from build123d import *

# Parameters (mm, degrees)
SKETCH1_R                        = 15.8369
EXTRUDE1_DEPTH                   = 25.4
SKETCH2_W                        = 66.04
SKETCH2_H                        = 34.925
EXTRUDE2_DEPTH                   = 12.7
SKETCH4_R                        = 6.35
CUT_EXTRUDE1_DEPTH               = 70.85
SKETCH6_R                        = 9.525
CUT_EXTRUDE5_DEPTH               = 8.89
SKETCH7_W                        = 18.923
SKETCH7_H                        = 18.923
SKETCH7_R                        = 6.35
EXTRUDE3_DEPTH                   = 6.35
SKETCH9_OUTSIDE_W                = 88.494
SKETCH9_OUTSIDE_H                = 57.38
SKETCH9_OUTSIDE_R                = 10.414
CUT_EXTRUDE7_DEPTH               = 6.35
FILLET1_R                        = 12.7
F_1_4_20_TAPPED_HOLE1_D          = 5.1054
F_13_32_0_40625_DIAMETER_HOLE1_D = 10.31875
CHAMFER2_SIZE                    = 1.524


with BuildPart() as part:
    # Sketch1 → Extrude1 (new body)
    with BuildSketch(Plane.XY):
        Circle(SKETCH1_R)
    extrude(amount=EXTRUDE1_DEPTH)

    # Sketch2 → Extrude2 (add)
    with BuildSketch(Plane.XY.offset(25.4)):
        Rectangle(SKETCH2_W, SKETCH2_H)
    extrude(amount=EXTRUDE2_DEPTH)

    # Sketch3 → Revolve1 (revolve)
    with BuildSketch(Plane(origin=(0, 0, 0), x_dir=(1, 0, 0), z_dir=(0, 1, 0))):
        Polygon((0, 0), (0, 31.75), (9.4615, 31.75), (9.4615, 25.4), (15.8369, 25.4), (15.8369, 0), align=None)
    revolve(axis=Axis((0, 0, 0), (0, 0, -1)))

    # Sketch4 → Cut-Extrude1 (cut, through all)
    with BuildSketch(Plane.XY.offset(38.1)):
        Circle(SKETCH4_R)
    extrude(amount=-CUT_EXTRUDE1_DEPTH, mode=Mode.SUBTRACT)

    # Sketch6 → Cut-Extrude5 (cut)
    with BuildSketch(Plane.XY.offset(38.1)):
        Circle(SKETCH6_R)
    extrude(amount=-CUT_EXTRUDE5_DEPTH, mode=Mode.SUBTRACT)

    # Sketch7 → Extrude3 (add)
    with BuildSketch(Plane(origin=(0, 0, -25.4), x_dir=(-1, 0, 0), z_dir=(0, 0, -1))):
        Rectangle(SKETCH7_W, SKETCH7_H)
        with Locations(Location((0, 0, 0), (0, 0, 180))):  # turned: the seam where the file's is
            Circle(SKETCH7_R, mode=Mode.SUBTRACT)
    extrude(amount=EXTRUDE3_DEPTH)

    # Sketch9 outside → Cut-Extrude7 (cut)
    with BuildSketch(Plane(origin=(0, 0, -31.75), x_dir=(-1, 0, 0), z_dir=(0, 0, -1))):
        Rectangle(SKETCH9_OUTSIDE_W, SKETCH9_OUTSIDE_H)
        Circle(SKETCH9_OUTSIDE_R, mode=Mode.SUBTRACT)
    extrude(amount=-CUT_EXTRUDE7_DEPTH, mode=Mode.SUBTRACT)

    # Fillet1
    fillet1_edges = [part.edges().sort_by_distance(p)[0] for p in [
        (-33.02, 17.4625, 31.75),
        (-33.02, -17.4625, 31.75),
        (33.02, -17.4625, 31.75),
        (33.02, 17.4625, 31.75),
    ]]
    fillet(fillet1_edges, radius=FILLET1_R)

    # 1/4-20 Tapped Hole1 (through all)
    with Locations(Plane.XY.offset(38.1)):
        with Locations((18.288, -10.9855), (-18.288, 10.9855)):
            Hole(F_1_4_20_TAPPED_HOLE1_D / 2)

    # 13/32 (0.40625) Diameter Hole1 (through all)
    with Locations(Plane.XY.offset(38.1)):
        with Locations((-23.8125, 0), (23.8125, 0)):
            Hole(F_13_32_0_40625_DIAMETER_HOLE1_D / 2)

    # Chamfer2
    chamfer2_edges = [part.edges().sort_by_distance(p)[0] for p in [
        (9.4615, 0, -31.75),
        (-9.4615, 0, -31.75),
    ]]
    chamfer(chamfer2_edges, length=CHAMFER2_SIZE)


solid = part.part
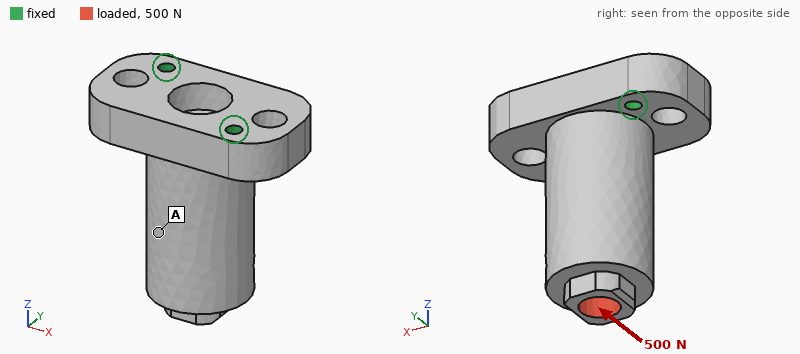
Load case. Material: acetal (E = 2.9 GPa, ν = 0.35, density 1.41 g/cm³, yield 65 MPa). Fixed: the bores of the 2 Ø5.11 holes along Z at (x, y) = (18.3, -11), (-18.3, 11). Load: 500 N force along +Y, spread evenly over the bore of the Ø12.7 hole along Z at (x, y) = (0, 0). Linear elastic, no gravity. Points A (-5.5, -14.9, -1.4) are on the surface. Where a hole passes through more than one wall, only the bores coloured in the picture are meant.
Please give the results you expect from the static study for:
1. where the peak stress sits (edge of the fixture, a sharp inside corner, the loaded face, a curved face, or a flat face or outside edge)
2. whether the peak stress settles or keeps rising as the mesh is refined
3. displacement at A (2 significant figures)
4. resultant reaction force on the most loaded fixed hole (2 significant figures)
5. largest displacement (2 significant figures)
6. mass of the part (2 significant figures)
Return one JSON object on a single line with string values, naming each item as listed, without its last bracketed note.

{"where the peak stress sits": "edge of the fixture", "whether the peak stress settles or keeps rising as the mesh is refined": "keeps rising", "displacement at A": "0.33 mm", "resultant reaction force on the most loaded fixed hole": "350 N", "largest displacement": "0.60 mm", "mass of the part": "80 g"}
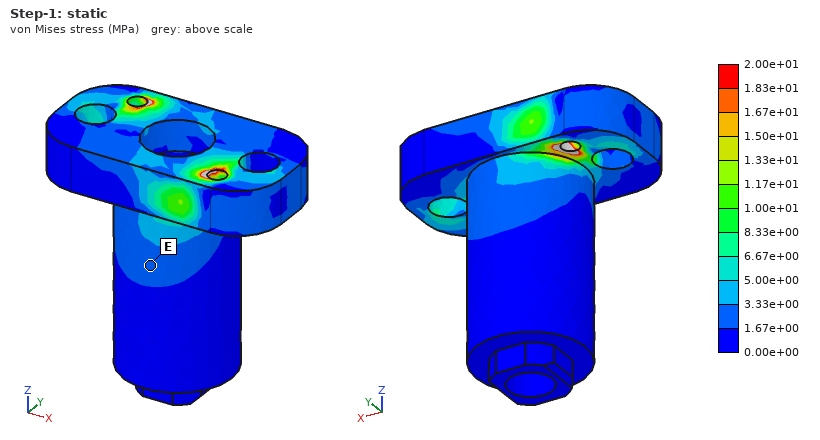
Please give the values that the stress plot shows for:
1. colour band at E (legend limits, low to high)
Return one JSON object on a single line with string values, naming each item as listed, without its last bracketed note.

{"colour band at E": "1.67e+00 to 3.33e+00 MPa"}
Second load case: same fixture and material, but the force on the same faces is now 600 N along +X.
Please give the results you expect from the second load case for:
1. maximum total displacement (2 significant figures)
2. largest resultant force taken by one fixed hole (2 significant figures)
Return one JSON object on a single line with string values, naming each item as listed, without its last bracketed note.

{"maximum total displacement": "0.46 mm", "largest resultant force taken by one fixed hole": "530 N"}
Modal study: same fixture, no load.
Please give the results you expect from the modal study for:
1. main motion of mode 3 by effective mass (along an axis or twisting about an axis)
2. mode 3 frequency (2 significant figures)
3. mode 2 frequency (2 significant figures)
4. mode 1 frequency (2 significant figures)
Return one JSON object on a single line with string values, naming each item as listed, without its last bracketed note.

{"main motion of mode 3 by effective mass": "along Z", "mode 3 frequency": "3100 Hz", "mode 2 frequency": "1500 Hz", "mode 1 frequency": "750 Hz"}
